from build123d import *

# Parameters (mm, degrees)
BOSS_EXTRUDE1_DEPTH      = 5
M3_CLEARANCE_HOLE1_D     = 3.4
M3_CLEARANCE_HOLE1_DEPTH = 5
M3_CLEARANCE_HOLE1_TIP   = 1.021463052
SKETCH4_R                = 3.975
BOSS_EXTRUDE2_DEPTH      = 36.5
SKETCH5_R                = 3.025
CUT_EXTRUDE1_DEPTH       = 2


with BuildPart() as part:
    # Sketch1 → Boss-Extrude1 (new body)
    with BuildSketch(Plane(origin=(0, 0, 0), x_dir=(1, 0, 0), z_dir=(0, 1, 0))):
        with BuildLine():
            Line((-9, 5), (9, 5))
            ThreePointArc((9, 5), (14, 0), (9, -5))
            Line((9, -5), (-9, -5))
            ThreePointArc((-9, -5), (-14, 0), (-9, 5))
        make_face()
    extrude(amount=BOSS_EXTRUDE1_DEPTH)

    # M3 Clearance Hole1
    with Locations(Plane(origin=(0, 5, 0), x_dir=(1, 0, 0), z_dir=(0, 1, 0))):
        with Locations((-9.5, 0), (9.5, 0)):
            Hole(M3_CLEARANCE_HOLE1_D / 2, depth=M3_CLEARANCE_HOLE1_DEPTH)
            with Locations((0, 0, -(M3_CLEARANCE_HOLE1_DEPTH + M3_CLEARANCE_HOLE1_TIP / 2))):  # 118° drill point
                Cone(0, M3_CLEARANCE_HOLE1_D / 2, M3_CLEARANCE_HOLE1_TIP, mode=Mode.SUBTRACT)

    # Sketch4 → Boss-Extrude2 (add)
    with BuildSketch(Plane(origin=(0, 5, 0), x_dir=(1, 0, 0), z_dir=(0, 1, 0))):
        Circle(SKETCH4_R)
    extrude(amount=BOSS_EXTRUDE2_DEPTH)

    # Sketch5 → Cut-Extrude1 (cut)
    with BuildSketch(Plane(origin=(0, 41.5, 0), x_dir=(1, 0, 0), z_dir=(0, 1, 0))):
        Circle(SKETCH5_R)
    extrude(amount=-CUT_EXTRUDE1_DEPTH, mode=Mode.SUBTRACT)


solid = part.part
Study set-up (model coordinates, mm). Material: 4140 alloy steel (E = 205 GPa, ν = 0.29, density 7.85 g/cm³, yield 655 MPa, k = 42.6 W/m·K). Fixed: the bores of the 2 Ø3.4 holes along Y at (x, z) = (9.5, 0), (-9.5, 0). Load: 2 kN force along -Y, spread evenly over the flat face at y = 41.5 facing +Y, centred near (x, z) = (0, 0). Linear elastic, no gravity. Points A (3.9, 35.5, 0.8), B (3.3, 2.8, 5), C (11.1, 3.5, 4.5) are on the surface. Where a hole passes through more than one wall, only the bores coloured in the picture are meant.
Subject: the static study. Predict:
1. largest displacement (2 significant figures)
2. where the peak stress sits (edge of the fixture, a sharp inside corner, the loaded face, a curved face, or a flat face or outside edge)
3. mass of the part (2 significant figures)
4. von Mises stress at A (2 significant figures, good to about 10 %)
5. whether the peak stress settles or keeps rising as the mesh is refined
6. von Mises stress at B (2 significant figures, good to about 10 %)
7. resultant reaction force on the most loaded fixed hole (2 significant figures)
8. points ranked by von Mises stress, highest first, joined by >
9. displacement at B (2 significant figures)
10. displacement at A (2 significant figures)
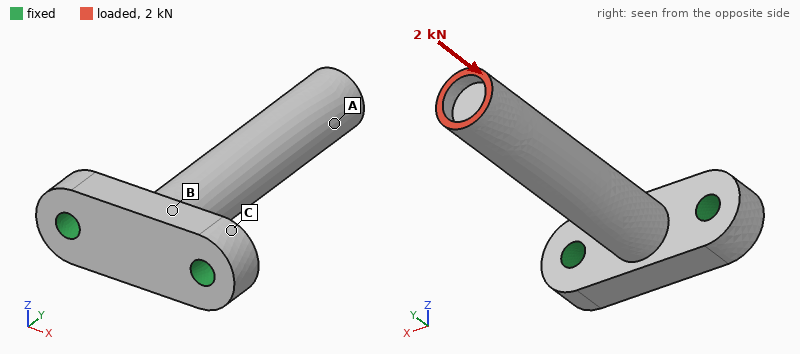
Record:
12 µm
edge of the fixture
23 g
44 MPa
keeps rising
32 MPa
1.0 kN
A > B > C
3.0 µm
9.6 µm
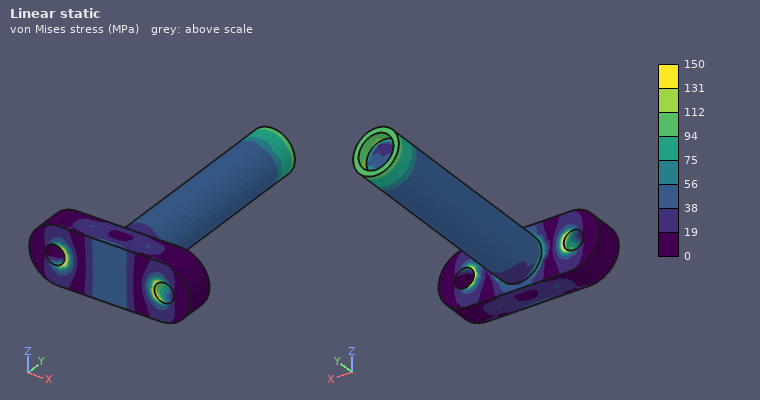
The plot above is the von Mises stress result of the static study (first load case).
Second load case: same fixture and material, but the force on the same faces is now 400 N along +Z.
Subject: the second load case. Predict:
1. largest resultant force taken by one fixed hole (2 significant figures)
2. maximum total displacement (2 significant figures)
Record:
200 N
0.27 mm
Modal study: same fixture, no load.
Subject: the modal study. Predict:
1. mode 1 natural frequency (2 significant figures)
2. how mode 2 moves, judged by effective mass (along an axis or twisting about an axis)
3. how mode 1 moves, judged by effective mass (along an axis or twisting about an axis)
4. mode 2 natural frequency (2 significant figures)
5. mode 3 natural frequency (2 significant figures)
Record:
3200 Hz
along X
along Z
3900 Hz
19 kHz
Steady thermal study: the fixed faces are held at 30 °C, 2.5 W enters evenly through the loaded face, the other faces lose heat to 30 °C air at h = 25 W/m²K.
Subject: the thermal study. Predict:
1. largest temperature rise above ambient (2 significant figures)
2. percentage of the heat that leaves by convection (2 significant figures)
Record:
45 K
23 %
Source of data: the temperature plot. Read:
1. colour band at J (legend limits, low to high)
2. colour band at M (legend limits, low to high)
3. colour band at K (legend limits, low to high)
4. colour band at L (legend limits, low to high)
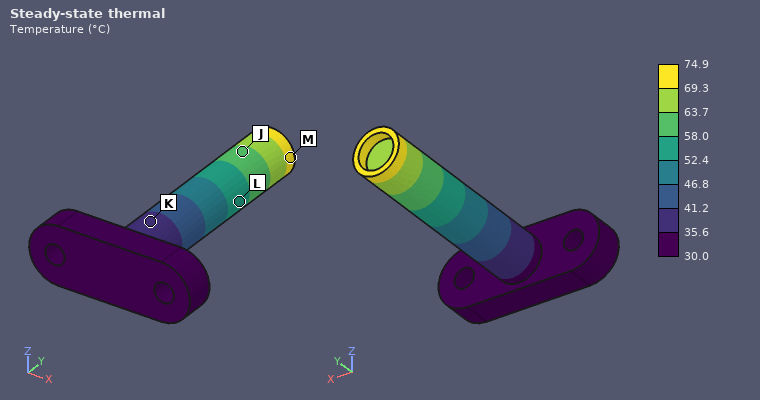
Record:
58.0 to 63.7 °C
69.3 to 74.9 °C
35.6 to 41.2 °C
52.4 to 58.0 °C
